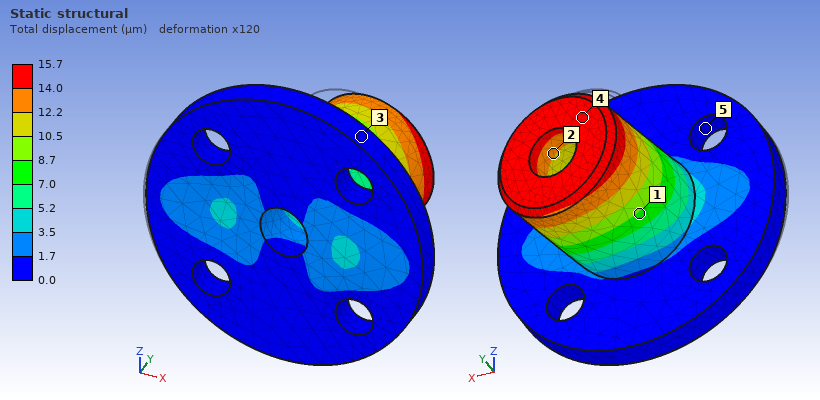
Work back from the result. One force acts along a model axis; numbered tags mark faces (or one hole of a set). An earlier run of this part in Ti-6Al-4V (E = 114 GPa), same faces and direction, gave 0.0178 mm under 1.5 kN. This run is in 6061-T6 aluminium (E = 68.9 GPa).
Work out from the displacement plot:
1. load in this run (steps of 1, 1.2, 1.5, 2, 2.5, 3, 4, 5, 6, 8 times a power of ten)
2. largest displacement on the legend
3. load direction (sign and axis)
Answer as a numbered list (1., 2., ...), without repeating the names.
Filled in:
1. 800 N
2. 15.7 µm
3. +X
